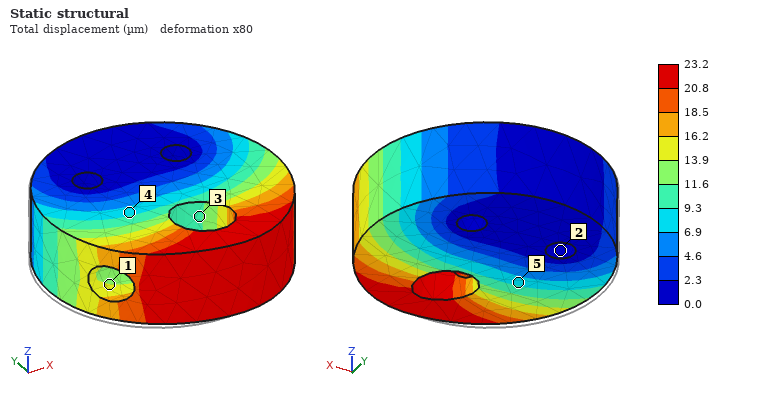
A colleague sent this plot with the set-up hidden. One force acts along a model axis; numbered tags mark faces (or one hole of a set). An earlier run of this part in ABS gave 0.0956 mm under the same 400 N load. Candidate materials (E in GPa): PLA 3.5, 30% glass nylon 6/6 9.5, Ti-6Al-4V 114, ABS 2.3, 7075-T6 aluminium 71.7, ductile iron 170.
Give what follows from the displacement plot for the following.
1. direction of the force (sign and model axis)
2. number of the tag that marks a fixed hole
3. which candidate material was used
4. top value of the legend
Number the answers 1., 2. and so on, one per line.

1. +X
2. 2
3. 30% glass nylon 6/6
4. 23.2 µm
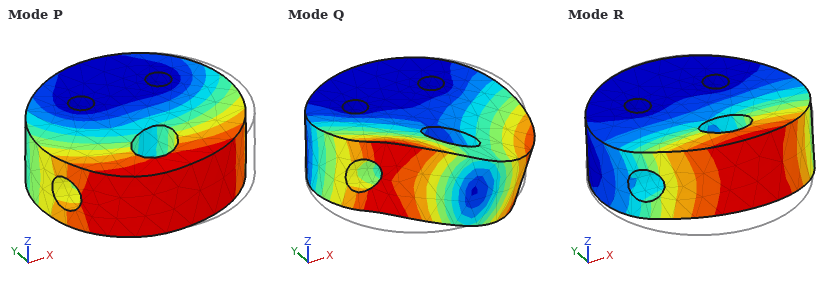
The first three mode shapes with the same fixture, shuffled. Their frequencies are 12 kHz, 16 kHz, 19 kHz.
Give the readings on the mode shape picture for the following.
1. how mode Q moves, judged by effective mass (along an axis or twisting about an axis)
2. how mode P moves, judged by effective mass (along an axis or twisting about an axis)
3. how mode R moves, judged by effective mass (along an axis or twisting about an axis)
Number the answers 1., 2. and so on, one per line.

1. twisting about Y
2. along X
3. along Z
